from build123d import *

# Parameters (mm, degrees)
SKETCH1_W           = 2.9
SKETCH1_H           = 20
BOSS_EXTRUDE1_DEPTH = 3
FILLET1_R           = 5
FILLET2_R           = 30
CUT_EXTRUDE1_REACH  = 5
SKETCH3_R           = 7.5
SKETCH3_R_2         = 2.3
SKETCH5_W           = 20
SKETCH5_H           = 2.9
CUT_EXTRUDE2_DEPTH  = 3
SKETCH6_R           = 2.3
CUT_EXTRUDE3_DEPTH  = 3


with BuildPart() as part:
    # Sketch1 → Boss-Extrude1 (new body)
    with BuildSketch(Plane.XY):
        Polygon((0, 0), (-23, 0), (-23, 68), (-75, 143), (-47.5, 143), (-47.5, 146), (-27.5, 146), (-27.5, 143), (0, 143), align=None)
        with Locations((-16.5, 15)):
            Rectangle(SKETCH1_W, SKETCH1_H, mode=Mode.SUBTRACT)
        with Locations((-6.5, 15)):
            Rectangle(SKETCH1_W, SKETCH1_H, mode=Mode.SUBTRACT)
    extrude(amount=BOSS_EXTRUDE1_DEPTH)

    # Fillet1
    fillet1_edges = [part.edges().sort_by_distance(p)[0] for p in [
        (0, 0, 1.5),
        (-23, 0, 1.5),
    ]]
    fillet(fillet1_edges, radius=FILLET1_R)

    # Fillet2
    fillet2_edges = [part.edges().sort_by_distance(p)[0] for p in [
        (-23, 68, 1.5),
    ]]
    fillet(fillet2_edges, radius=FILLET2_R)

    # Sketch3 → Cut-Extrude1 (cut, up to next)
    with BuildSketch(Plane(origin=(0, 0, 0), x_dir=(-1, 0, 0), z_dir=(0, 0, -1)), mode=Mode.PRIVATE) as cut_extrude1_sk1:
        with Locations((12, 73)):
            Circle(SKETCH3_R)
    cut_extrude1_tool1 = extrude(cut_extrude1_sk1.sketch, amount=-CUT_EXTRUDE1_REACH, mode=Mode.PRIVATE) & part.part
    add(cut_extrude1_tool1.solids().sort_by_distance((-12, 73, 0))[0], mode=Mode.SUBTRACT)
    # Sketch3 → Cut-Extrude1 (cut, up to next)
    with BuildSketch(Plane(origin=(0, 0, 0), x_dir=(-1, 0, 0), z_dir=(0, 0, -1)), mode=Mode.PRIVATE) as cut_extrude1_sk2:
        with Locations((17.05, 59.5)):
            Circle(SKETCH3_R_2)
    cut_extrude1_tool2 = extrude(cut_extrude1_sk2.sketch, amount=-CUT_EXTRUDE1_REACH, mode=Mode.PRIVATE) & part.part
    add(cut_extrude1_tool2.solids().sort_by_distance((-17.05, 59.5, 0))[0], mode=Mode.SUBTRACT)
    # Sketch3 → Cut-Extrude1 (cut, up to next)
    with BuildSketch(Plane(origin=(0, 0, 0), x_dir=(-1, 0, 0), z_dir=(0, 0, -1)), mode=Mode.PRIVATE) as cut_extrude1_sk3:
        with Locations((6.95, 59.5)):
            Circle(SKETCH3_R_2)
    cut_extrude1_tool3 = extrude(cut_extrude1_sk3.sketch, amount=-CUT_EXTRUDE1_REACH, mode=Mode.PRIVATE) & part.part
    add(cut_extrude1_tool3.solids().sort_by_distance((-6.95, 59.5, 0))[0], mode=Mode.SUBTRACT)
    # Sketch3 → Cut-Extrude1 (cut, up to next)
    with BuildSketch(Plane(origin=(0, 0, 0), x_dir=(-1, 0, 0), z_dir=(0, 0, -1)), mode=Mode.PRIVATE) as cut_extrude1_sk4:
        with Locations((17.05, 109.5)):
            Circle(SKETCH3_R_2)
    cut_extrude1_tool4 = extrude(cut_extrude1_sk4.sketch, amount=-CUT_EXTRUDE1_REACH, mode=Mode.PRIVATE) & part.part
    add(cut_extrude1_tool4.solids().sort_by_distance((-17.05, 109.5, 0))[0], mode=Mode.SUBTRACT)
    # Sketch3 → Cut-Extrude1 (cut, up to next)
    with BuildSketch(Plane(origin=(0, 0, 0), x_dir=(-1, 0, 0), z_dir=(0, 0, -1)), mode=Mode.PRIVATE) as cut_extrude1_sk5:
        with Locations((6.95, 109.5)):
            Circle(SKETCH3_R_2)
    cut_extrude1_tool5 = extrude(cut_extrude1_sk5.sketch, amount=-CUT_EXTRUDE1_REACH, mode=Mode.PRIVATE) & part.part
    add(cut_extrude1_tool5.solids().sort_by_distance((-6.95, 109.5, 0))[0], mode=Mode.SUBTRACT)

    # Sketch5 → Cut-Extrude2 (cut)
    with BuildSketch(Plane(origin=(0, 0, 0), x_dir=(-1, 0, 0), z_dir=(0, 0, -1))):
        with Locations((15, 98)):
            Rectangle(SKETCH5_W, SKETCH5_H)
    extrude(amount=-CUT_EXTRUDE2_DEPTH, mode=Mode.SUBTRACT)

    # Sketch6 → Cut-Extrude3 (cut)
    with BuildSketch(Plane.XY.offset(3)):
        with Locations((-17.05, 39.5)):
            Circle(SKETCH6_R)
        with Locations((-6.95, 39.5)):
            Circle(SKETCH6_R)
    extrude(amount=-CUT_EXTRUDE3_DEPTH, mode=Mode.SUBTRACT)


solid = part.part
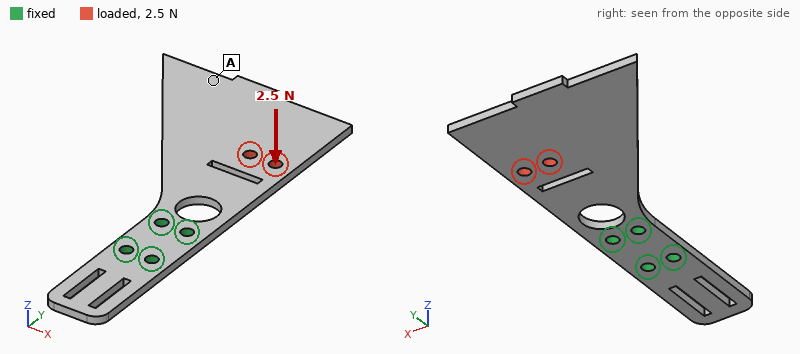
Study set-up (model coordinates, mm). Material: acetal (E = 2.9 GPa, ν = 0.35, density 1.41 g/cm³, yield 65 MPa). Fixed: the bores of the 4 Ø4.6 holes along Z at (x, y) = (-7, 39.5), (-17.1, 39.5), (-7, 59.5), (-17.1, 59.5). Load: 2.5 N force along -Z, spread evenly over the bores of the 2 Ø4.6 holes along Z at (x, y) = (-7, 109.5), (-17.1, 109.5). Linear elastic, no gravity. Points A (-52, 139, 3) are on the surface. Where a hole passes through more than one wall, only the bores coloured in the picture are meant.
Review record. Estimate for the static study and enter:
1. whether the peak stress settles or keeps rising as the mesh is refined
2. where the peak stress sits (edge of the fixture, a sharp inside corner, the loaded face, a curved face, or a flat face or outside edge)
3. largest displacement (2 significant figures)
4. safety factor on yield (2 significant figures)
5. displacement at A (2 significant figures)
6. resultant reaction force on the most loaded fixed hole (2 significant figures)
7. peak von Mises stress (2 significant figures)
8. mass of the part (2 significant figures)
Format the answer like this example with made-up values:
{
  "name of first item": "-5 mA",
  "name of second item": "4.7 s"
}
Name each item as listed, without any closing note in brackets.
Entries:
{
  "whether the peak stress settles or keeps rising as the mesh is refined": "settles",
  "where the peak stress sits": "a curved face",
  "largest displacement": "2.0 mm",
  "safety factor on yield": "9.0",
  "displacement at A": "1.8 mm",
  "resultant reaction force on the most loaded fixed hole": "1.3 N",
  "peak von Mises stress": "7.2 MPa",
  "mass of the part": "21 g"
}
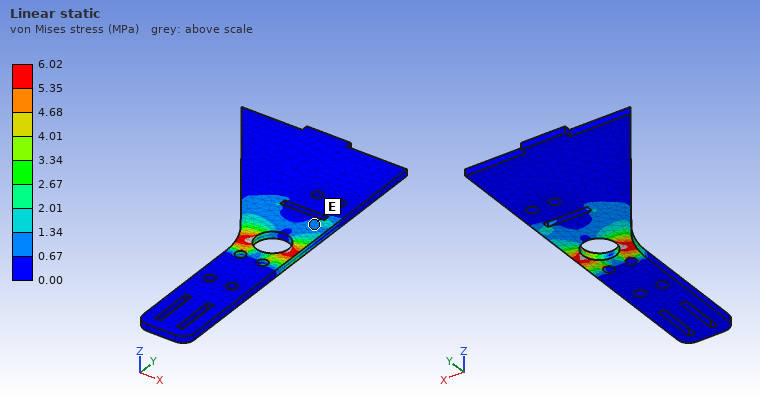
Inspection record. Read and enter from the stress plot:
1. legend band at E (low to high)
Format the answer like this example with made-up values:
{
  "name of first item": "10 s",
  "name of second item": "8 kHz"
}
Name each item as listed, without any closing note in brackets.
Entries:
{
  "legend band at E": "0.67 to 1.34 MPa"
}
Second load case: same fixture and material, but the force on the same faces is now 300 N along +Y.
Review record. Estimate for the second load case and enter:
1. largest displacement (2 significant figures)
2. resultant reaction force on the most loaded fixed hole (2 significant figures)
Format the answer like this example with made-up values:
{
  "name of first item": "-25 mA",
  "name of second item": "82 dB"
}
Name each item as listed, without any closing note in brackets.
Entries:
{
  "largest displacement": "0.22 mm",
  "resultant reaction force on the most loaded fixed hole": "140 N"
}
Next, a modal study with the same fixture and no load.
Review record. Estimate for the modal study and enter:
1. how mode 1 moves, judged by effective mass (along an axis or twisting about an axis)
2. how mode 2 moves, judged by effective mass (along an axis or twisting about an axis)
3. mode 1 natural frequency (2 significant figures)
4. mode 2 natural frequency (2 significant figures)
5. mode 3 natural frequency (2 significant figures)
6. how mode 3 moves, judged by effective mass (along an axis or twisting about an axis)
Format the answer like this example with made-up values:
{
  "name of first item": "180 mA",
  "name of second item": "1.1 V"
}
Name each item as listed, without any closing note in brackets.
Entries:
{
  "how mode 1 moves, judged by effective mass": "along Z",
  "how mode 2 moves, judged by effective mass": "twisting about Y",
  "mode 1 natural frequency": "49 Hz",
  "mode 2 natural frequency": "180 Hz",
  "mode 3 natural frequency": "360 Hz",
  "how mode 3 moves, judged by effective mass": "along X"
}
